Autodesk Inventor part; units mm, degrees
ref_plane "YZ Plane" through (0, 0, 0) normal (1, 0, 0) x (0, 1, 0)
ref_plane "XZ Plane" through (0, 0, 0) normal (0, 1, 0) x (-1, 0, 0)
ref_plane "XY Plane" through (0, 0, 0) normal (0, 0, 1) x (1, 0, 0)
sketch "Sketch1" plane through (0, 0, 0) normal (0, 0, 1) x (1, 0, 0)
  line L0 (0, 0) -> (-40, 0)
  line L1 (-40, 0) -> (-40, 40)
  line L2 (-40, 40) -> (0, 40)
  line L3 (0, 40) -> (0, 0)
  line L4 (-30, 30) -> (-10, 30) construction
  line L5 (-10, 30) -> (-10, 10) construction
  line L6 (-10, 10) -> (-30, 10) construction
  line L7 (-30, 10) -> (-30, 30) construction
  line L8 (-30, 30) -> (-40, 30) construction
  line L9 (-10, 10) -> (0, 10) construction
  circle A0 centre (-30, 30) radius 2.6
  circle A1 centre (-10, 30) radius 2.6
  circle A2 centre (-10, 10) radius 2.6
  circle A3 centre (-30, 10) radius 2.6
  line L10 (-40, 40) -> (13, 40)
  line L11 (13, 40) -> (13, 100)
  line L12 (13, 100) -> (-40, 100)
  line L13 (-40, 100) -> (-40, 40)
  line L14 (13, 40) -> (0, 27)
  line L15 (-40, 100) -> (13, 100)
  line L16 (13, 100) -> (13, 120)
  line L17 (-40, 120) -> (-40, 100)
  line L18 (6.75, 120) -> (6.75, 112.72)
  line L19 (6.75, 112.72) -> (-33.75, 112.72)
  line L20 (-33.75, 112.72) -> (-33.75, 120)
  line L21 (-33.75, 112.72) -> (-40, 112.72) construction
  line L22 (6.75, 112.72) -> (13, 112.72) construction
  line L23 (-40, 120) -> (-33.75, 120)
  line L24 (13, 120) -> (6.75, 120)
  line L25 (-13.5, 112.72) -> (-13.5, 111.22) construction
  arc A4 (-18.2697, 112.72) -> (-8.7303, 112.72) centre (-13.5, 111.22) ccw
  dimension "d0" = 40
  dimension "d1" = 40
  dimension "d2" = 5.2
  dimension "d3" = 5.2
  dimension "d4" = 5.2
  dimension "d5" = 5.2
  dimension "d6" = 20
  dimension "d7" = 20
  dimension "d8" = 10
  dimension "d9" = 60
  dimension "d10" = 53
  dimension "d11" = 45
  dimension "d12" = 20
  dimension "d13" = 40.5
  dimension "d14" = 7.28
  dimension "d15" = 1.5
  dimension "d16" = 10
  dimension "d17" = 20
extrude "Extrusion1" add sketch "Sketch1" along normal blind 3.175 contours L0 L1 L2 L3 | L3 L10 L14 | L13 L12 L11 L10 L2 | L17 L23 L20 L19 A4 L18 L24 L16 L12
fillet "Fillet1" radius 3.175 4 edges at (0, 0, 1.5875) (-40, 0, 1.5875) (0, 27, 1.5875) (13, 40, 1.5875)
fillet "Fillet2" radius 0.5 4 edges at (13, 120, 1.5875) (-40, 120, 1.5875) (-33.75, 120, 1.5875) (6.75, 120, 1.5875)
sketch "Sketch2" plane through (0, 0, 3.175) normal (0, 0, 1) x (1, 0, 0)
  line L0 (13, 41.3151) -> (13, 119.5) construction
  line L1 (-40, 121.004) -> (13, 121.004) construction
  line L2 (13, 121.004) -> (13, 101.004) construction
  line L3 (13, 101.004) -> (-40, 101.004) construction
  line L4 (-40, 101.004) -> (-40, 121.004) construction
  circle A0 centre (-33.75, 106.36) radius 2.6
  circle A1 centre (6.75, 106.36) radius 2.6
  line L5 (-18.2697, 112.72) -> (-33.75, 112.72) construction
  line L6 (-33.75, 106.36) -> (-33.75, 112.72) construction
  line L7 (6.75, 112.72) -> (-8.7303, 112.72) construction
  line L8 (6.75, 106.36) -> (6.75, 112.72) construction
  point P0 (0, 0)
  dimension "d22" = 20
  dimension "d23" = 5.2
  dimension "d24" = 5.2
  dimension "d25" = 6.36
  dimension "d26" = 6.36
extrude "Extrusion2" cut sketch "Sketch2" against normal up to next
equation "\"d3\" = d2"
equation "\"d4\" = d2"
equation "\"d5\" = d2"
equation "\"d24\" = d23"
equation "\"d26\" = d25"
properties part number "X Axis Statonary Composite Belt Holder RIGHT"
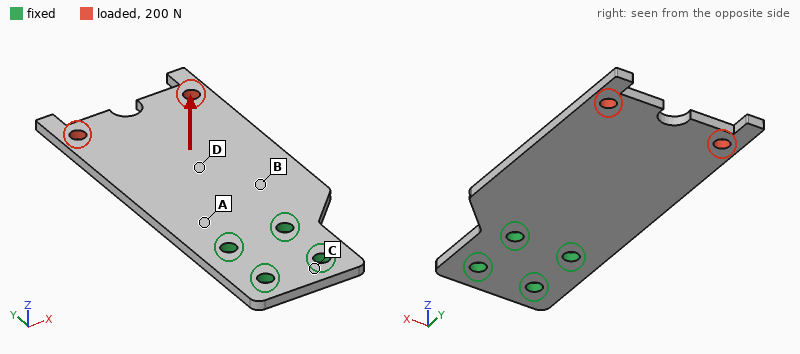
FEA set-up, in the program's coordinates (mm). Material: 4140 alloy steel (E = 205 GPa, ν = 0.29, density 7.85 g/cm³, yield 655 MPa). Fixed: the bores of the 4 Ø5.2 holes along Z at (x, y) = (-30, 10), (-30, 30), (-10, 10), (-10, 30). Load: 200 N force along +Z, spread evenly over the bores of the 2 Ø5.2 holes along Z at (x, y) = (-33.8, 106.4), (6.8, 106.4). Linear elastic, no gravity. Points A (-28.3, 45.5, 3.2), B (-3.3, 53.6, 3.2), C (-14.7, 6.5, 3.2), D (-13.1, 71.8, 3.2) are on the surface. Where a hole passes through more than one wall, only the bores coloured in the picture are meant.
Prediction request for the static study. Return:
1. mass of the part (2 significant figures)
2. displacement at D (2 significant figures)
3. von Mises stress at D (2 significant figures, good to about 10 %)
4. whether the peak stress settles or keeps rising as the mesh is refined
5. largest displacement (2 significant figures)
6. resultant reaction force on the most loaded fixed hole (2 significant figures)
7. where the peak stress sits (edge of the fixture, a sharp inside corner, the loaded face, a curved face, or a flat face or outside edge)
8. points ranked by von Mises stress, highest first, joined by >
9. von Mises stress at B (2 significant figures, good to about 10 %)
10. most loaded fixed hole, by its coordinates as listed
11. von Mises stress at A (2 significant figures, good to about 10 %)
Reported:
140 g
0.39 mm
71 MPa
keeps rising
1.3 mm
240 N
edge of the fixture
A > B > D > C
110 MPa
(-10, 30)
140 MPa
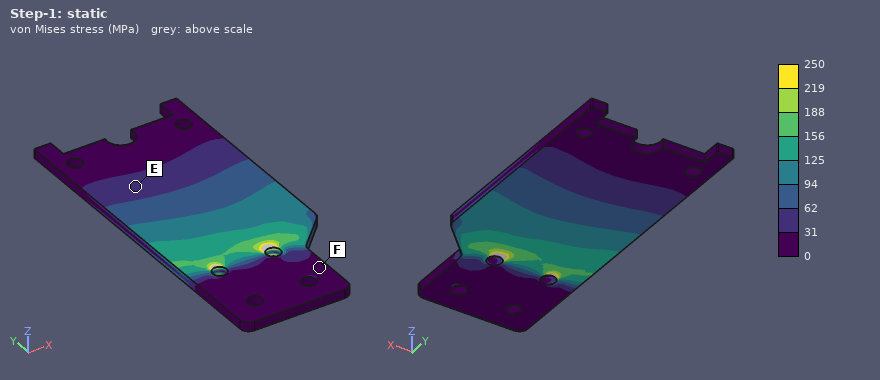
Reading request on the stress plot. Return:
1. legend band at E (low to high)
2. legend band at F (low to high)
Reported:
31 to 62 MPa
0 to 31 MPa
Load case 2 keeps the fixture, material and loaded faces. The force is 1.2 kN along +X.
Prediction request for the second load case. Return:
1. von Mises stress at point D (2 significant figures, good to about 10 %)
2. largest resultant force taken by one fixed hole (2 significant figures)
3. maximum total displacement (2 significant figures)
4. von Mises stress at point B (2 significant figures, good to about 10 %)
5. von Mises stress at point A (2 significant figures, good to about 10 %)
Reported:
19 MPa
3.1 kN
65 µm
27 MPa
45 MPa
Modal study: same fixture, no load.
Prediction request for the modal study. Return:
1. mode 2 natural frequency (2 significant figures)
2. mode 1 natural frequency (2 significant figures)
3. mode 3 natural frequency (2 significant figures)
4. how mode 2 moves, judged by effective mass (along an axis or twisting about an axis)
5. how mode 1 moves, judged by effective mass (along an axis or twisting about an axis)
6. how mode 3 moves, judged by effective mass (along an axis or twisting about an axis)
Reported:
1200 Hz
380 Hz
2300 Hz
twisting about Y
along Z
along Z
